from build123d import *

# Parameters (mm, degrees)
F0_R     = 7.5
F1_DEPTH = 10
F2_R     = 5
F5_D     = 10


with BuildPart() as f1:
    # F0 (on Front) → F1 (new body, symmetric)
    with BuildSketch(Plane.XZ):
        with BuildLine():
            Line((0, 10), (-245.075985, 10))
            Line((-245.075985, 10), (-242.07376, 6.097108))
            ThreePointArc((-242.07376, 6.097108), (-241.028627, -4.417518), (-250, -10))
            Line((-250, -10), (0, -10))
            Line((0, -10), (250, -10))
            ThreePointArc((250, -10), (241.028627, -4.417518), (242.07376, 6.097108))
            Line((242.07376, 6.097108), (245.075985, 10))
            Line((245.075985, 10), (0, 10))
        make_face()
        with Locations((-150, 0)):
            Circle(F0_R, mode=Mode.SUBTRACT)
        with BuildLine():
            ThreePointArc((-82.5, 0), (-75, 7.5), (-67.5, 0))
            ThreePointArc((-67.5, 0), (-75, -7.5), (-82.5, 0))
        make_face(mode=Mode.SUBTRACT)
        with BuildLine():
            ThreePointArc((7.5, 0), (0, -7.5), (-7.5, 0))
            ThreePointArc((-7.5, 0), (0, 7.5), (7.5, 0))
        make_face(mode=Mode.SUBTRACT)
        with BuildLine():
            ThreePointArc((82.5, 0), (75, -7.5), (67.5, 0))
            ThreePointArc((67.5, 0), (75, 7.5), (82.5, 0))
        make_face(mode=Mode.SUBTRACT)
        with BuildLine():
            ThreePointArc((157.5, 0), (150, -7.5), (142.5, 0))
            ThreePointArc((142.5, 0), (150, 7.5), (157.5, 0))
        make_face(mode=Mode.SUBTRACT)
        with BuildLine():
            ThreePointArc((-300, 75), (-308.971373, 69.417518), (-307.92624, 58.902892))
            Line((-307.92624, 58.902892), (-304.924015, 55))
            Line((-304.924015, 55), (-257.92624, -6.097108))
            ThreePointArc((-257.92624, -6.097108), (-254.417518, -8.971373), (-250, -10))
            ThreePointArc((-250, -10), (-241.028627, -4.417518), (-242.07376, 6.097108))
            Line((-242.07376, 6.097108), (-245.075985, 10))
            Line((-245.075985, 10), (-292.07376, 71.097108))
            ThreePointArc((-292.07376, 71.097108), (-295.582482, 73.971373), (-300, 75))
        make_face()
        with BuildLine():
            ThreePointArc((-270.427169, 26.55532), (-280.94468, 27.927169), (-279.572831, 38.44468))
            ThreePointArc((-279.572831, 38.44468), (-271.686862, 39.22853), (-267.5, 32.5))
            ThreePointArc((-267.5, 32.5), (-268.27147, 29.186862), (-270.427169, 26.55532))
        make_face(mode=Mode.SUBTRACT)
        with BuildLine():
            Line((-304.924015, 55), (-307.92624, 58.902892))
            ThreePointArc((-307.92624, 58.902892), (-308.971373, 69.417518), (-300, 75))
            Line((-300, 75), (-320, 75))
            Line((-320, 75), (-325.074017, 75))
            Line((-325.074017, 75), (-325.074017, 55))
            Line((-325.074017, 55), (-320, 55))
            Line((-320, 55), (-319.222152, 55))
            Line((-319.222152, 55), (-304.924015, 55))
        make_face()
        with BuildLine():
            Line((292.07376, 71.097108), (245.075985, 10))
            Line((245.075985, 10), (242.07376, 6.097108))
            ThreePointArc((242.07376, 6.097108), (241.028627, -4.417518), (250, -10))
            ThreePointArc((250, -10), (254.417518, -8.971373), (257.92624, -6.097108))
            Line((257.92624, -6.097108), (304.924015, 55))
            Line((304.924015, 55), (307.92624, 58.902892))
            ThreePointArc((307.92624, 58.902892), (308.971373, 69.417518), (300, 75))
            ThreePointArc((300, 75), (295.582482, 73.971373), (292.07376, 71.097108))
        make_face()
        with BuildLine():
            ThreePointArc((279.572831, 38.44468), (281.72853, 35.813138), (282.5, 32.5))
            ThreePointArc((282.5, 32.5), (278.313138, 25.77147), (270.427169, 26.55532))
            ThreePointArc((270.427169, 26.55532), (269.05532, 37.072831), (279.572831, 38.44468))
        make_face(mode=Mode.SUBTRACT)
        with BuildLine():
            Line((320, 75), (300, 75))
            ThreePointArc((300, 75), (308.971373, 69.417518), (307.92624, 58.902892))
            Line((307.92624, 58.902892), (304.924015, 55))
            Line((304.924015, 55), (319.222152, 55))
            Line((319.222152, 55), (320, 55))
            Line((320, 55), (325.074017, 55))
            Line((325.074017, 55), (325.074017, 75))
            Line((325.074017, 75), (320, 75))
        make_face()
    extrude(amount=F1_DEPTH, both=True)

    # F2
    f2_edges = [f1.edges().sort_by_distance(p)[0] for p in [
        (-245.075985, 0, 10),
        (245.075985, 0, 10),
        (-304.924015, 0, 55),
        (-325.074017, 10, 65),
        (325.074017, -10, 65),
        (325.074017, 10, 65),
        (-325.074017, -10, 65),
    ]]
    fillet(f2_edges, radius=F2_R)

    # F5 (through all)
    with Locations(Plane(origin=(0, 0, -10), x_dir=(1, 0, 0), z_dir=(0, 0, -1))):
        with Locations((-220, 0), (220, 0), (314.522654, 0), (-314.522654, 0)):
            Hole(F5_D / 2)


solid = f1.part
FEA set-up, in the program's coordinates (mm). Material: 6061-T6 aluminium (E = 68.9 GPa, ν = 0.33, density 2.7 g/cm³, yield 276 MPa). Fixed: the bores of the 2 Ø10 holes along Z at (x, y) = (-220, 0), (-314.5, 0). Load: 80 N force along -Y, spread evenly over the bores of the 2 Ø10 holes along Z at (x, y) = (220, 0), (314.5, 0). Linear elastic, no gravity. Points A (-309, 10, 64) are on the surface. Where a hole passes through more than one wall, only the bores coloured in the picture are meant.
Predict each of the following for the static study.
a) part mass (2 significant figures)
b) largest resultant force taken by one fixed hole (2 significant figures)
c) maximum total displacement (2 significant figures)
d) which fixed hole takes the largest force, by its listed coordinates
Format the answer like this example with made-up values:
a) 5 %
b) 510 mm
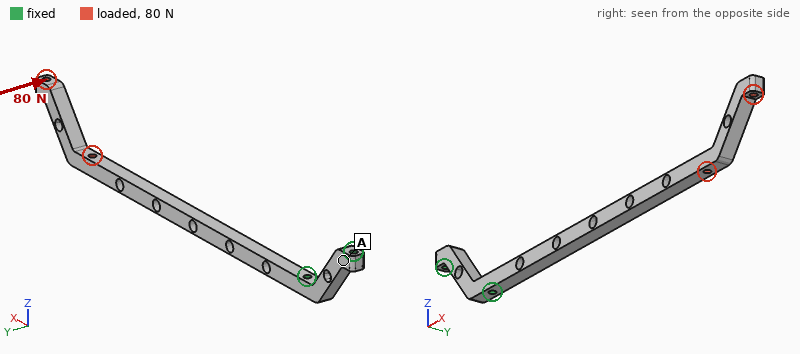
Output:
a) 690 g
b) 110 N
c) 6.3 mm
d) (-220, 0)
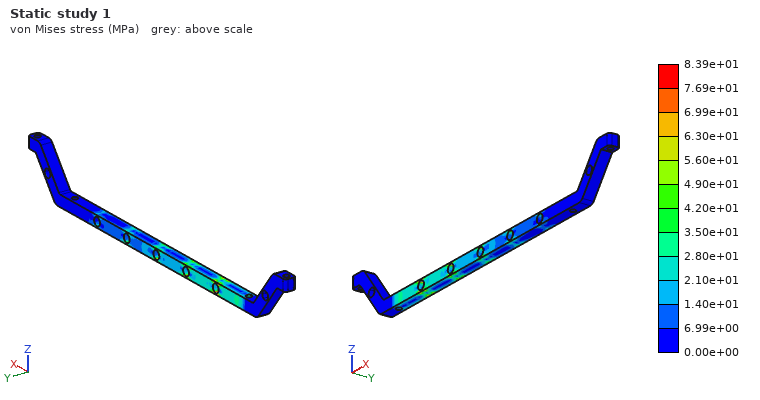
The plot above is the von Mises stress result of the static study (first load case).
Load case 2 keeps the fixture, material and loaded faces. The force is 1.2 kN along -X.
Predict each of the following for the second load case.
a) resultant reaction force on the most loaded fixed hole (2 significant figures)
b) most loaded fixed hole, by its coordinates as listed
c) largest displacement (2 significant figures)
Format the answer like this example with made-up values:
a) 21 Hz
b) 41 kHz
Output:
a) 1.2 kN
b) (-220, 0)
c) 7.3 mm
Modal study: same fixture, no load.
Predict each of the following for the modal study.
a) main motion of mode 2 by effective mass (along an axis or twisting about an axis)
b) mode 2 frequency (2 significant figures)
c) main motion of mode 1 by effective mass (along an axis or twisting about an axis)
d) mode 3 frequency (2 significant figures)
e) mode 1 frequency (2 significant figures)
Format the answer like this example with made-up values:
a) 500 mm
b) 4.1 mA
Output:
a) along Z
b) 51 Hz
c) along Y
d) 260 Hz
e) 43 Hz
